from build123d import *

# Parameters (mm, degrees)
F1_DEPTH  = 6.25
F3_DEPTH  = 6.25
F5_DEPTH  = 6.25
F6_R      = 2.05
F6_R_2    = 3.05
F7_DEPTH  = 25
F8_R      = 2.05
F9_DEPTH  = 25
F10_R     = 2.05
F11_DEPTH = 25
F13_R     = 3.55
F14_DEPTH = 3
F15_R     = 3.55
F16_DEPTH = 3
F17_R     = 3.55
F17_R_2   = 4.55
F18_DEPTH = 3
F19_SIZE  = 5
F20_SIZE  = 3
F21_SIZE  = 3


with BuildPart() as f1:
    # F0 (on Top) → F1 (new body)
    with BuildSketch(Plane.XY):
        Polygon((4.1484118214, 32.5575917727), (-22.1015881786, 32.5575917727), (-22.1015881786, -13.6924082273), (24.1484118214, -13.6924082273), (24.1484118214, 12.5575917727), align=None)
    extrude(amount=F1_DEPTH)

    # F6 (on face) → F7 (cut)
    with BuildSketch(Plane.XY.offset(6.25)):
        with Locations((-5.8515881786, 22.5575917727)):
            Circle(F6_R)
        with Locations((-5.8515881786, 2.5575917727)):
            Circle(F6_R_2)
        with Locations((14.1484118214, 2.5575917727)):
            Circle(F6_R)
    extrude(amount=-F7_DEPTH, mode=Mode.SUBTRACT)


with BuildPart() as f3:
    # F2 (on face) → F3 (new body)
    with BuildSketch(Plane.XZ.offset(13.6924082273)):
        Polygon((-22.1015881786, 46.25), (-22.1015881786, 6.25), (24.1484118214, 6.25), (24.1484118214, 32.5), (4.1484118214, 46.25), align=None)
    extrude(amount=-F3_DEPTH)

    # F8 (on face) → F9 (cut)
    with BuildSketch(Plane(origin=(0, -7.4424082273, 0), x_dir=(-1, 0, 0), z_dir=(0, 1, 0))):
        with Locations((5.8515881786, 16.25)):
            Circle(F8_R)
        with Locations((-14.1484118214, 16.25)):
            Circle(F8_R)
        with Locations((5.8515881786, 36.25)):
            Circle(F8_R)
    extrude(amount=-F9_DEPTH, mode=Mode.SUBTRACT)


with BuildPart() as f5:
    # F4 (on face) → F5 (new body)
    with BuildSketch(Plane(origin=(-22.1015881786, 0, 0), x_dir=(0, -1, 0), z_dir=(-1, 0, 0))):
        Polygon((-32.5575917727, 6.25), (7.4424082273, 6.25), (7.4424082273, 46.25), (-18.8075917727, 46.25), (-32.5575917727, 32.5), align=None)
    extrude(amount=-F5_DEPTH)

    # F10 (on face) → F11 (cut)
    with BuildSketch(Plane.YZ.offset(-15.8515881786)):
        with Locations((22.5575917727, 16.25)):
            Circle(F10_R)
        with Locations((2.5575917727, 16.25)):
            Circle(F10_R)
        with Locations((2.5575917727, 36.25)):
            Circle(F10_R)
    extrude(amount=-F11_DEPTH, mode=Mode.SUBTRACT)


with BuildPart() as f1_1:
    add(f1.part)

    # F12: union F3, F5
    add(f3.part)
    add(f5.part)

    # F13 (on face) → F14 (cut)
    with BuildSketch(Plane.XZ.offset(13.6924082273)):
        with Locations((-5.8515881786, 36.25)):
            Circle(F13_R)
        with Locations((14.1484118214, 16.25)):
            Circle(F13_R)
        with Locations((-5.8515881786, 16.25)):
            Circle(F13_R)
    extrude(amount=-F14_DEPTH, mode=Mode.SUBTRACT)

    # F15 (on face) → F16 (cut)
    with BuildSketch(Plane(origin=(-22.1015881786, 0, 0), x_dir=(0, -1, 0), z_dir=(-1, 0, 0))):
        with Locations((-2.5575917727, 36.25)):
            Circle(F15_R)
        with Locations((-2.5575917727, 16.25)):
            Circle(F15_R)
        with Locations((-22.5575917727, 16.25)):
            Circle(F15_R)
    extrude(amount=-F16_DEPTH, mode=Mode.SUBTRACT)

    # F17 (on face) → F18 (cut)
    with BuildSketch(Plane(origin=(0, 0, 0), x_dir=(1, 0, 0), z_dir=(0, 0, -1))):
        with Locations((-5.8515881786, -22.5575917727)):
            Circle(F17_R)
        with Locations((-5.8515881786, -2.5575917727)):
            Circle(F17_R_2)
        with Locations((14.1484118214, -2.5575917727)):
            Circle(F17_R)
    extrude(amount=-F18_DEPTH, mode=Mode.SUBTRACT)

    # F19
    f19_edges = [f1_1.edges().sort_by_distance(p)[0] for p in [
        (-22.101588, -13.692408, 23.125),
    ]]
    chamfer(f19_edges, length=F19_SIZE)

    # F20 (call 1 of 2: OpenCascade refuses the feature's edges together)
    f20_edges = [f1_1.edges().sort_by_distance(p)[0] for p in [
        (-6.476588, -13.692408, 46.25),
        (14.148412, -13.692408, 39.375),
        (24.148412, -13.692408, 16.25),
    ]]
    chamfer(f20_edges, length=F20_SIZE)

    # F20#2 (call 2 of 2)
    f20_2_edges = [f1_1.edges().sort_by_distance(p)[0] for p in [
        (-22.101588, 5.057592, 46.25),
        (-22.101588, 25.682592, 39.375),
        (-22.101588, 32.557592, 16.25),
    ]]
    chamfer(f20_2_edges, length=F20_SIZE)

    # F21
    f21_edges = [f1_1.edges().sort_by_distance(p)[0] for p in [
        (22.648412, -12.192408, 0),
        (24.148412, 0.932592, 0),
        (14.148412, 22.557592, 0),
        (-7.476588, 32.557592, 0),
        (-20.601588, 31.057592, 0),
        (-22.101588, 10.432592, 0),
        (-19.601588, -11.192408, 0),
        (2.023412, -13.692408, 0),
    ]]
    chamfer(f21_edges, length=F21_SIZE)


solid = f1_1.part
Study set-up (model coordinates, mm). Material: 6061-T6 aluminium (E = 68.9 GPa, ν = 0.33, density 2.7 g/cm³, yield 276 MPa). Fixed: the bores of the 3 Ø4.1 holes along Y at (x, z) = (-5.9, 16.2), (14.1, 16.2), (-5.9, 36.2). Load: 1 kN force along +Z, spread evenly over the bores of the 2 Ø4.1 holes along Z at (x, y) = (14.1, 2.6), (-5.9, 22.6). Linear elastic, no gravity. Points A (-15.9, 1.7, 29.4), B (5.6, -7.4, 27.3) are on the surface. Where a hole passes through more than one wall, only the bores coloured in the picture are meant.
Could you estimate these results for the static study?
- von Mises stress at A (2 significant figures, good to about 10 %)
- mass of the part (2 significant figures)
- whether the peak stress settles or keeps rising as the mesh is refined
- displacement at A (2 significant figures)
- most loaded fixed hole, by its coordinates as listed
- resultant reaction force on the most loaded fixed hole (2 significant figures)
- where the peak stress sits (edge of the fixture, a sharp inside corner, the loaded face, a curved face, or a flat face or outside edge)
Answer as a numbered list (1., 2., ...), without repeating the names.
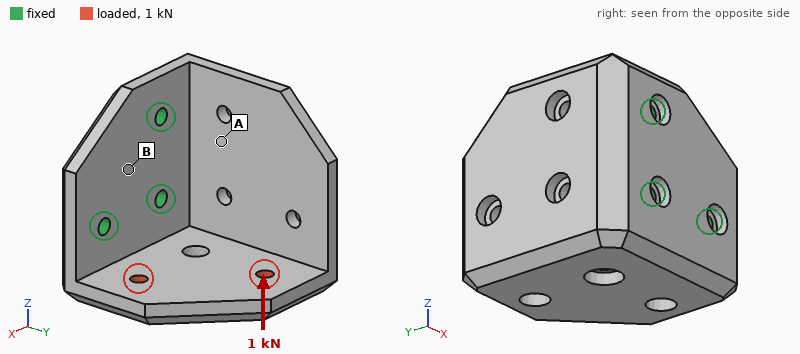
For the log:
1. 16 MPa
2. 77 g
3. keeps rising
4. 0.024 mm
5. (-5.9, 16.2)
6. 1.0 kN
7. edge of the fixture
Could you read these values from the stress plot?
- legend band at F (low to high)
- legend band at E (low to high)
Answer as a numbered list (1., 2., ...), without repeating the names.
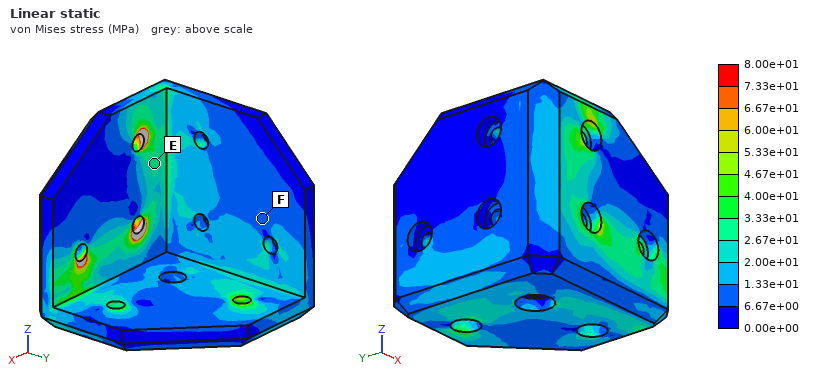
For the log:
1. 6.67e+00 to 1.33e+01 MPa
2. 2.67e+01 to 3.33e+01 MPa
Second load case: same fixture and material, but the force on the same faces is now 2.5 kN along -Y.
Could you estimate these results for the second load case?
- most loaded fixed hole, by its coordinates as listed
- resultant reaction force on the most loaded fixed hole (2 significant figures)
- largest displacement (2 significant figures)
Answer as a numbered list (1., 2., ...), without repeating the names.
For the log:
1. (-5.9, 16.2)
2. 2.1 kN
3. 89 µm
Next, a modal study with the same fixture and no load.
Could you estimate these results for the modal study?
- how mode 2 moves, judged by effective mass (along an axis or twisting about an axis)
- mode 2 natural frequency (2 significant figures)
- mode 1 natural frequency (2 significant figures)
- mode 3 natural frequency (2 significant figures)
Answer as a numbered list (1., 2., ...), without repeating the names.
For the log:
1. along Z
2. 3000 Hz
3. 2900 Hz
4. 6500 Hz
